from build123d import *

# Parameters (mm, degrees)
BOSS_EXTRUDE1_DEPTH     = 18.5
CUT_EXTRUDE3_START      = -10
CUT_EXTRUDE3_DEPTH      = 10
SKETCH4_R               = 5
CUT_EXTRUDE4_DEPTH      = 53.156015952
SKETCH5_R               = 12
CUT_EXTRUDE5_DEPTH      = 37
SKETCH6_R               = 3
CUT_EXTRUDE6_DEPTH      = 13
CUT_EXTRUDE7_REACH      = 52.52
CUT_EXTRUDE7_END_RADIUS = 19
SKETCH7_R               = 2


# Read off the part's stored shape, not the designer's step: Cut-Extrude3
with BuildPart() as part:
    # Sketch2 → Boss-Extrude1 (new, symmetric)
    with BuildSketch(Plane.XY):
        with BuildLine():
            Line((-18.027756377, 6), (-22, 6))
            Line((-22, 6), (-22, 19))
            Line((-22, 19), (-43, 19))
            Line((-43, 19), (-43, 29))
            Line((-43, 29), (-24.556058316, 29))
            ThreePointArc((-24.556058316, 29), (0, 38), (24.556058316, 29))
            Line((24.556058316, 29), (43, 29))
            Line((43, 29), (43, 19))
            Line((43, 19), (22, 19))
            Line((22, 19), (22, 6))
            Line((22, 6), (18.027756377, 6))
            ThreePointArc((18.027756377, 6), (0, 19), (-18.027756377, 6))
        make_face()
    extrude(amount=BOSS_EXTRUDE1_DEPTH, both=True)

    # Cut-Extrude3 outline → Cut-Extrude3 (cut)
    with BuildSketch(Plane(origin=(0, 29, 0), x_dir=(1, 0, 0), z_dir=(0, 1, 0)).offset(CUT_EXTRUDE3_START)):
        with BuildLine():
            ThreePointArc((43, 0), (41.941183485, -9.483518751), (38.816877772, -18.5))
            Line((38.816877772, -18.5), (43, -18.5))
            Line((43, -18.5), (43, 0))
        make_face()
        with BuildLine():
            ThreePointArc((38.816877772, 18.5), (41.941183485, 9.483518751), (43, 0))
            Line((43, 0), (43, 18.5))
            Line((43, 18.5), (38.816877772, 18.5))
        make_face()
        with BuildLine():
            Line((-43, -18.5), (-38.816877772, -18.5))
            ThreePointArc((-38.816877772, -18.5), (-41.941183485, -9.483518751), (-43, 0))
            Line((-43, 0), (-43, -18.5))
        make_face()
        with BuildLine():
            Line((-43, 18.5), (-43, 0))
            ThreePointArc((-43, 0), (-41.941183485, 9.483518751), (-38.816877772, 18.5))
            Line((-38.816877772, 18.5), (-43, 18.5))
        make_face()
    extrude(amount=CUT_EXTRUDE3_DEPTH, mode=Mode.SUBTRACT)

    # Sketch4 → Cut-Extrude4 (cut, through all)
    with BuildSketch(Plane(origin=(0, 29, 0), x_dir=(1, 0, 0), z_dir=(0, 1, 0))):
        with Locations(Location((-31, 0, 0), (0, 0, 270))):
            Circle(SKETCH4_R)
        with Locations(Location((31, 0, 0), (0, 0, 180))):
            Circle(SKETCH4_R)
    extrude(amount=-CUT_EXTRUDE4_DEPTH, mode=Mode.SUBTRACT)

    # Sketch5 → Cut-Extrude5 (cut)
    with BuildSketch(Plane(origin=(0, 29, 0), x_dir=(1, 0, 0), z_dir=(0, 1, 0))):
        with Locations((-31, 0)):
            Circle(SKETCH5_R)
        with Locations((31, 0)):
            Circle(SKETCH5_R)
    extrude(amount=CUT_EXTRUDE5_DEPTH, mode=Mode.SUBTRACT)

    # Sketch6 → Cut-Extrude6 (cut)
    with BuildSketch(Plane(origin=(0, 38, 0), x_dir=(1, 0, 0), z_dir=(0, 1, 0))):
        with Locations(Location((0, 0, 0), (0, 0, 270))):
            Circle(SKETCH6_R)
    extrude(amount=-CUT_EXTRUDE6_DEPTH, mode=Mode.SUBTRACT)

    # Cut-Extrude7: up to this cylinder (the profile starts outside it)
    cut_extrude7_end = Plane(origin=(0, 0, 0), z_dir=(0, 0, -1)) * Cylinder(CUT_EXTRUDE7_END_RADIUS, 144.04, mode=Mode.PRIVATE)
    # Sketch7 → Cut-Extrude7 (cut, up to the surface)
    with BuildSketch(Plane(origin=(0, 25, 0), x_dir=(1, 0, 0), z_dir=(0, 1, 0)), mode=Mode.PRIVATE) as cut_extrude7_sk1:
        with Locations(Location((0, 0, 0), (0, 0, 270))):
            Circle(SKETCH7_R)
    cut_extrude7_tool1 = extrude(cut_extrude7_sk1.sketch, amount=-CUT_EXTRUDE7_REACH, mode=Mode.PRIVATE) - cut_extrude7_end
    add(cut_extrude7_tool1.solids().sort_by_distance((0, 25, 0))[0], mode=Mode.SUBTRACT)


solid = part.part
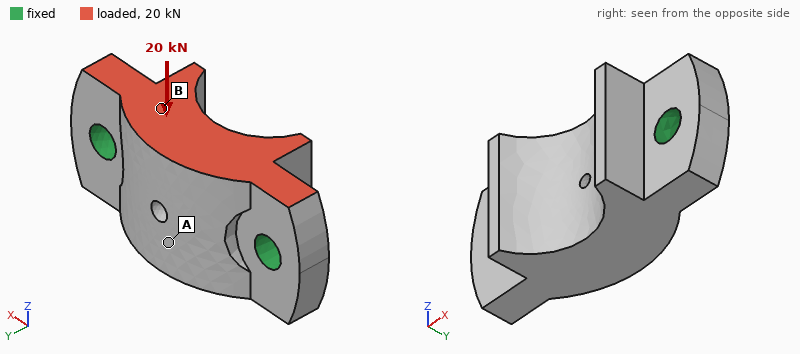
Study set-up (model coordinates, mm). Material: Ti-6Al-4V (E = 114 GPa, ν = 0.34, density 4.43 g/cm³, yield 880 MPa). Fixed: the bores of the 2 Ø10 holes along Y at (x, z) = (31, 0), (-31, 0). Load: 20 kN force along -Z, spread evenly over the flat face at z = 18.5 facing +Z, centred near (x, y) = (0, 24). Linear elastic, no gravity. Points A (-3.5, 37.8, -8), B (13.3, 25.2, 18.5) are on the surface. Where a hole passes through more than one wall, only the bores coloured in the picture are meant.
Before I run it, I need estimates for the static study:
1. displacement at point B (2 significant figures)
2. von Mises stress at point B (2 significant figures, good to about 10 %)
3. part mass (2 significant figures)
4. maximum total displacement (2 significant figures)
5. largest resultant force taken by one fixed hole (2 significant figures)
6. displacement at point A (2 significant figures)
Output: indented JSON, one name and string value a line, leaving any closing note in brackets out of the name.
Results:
{
  "displacement at point B": "12 µm",
  "von Mises stress at point B": "32 MPa",
  "part mass": "210 g",
  "maximum total displacement": "17 µm",
  "largest resultant force taken by one fixed hole": "10 kN",
  "displacement at point A": "13 µm"
}
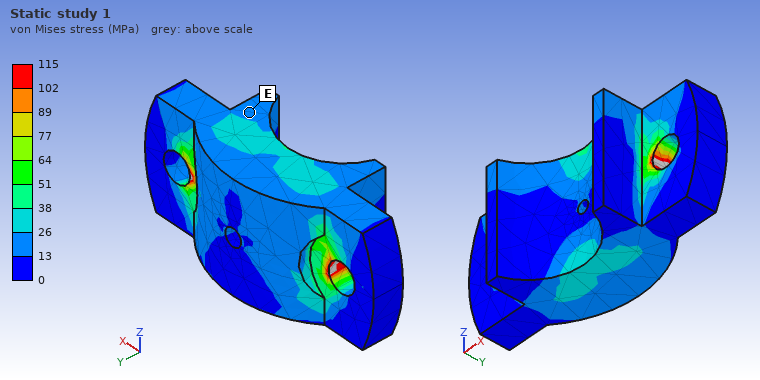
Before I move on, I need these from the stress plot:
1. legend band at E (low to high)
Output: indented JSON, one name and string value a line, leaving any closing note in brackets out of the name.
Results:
{
  "legend band at E": "13 to 26 MPa"
}
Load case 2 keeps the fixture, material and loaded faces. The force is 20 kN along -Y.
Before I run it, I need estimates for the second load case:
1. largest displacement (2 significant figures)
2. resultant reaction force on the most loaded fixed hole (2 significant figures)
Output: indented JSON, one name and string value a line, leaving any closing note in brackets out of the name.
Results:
{
  "largest displacement": "98 µm",
  "resultant reaction force on the most loaded fixed hole": "10 kN"
}
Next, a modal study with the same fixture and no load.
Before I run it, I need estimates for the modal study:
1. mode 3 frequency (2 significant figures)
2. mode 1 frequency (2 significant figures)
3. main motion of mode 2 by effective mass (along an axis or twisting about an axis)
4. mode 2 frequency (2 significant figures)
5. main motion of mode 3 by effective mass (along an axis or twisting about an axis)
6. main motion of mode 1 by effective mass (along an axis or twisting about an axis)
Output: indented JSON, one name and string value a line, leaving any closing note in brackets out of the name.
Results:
{
  "mode 3 frequency": "15 kHz",
  "mode 1 frequency": "9900 Hz",
  "main motion of mode 2 by effective mass": "along Y",
  "mode 2 frequency": "12 kHz",
  "main motion of mode 3 by effective mass": "along Z",
  "main motion of mode 1 by effective mass": "twisting about X"
}
